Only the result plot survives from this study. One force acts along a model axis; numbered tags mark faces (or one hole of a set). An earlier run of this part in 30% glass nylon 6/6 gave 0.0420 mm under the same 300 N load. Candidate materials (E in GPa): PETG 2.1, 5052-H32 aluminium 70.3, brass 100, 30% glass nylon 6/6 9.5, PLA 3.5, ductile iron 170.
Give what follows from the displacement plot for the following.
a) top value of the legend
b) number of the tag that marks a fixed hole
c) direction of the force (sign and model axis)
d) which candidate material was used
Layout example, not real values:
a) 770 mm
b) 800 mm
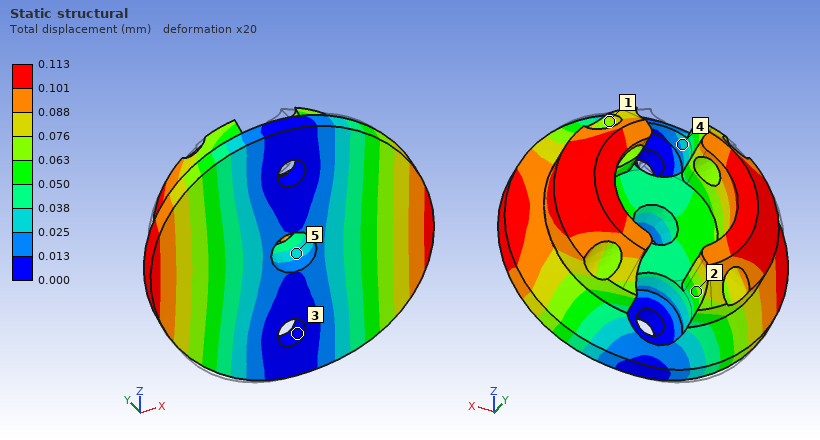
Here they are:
a) 0.113 mm
b) 3
c) +X
d) PLA
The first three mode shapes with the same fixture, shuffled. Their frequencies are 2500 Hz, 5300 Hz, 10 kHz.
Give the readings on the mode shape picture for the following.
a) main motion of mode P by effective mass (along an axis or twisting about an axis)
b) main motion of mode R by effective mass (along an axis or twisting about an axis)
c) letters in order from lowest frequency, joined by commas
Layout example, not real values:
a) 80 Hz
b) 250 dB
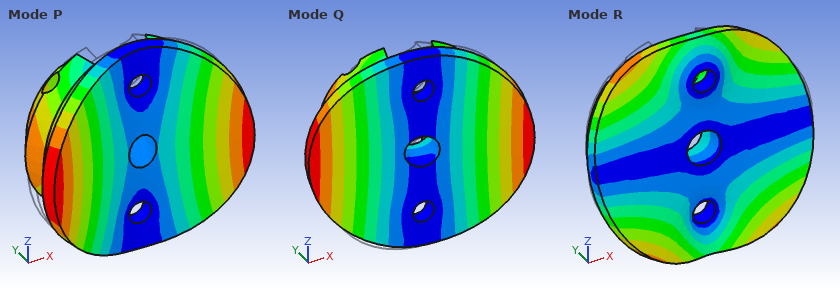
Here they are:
a) along Y
b) along Z
c) Q, P, R
